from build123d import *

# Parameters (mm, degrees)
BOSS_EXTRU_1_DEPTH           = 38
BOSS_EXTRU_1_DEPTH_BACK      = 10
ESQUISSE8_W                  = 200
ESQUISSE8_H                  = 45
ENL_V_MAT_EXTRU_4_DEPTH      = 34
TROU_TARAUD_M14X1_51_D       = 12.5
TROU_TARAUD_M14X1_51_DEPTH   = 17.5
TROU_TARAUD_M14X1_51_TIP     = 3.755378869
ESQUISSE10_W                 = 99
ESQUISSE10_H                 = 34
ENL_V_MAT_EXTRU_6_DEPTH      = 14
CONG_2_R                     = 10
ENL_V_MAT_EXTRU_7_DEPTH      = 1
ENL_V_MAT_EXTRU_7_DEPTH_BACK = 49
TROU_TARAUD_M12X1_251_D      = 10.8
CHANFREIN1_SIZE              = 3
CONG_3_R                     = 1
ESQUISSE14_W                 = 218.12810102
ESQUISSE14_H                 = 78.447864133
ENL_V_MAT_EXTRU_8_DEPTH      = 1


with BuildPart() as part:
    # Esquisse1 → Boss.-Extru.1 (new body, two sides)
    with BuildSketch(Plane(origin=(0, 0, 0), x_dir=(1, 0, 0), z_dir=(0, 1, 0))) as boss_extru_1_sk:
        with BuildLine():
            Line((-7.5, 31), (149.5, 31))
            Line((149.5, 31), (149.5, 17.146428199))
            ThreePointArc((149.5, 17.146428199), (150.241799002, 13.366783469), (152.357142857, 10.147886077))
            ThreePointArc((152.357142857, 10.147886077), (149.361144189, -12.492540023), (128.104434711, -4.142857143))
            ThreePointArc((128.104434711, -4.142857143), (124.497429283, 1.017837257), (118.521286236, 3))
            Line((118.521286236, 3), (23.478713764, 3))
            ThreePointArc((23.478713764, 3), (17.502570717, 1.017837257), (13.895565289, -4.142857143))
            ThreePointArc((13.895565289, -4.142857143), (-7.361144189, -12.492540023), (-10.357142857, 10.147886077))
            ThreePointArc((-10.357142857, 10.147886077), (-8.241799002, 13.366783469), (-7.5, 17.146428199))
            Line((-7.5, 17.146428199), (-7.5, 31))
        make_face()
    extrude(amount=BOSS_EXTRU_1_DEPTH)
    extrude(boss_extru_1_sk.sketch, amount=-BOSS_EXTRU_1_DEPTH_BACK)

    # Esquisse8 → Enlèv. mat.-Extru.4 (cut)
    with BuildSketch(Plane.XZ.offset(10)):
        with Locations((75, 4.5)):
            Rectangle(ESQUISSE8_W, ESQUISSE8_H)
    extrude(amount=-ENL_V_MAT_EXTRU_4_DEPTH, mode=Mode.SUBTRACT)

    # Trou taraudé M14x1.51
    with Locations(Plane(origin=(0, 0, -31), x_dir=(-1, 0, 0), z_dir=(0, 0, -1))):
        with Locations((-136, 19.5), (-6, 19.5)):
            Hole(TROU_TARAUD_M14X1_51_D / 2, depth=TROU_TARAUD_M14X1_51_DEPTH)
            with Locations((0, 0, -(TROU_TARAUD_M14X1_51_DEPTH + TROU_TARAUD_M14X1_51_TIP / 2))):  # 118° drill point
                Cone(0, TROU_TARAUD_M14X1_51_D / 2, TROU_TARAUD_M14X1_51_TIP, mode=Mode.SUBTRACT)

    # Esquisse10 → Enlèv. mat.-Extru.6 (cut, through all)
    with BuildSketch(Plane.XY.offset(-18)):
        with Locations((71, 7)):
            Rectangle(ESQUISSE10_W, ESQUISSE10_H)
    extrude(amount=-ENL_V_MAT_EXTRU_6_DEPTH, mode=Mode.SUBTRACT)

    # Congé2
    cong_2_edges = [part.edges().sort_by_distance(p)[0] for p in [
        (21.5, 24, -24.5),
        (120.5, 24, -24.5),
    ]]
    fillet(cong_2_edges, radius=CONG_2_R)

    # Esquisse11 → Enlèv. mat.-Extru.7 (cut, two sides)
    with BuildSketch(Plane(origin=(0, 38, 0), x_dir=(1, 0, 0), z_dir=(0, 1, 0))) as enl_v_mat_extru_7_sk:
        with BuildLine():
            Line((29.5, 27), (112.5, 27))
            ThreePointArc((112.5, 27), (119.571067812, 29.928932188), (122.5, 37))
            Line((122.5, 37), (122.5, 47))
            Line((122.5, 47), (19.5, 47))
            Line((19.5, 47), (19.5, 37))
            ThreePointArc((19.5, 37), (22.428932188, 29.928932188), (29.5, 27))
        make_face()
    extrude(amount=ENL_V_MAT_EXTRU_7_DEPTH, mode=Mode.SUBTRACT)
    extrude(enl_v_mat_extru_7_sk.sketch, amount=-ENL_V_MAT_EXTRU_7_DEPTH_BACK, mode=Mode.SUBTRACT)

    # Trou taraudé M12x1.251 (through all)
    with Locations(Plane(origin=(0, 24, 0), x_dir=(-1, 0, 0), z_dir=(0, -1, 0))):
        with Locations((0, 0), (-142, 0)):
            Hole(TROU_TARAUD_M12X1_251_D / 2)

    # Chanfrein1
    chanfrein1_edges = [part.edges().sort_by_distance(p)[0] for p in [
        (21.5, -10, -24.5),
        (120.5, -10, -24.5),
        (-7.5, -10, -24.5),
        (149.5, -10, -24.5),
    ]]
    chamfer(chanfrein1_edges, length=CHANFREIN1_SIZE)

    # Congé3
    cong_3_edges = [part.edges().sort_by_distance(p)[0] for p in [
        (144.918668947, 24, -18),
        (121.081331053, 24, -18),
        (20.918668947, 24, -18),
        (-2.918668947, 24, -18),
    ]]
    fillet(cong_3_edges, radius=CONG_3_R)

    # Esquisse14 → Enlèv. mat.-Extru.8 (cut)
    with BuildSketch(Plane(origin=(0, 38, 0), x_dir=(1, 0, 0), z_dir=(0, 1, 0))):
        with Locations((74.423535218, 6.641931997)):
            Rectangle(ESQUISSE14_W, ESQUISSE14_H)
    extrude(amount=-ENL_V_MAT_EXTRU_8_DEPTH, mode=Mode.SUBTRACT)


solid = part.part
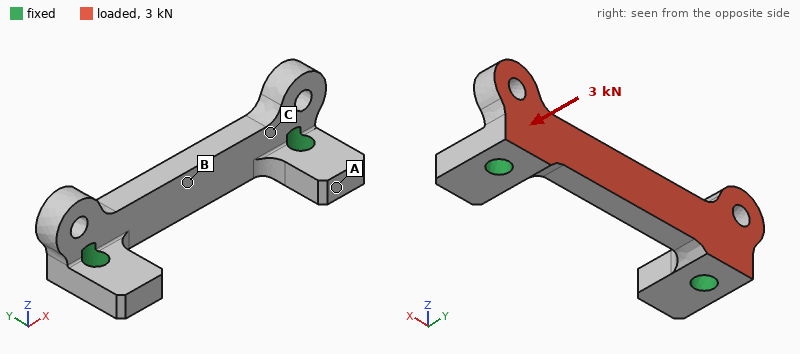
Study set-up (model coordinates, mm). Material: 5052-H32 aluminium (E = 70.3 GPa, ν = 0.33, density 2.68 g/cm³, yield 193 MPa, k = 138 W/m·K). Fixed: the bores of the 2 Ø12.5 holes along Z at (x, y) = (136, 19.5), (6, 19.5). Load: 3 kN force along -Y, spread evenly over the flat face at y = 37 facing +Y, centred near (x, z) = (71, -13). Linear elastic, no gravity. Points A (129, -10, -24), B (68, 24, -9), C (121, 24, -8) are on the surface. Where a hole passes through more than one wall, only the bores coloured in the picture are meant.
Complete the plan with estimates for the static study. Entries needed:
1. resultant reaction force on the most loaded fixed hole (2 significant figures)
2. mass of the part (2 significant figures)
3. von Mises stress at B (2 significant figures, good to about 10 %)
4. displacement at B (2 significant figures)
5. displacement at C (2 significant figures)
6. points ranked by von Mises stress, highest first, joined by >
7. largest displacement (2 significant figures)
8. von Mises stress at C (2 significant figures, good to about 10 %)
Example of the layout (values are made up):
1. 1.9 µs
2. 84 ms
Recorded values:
1. 1.6 kN
2. 230 g
3. 11 MPa
4. 28 µm
5. 7.6 µm
6. B > C > A
7. 31 µm
8. 7.2 MPa
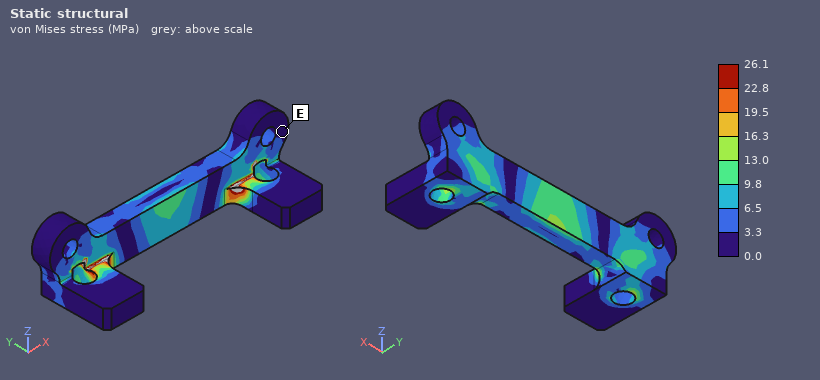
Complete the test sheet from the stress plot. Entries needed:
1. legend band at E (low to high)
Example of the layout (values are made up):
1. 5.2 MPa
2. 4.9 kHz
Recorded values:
1. 0.0 to 3.3 MPa
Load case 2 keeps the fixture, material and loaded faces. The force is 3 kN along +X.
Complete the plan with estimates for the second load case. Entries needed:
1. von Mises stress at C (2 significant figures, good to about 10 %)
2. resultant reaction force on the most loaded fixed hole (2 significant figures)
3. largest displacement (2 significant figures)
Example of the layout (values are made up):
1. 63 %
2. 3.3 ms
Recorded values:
1. 3.5 MPa
2. 1.5 kN
3. 7.5 µm
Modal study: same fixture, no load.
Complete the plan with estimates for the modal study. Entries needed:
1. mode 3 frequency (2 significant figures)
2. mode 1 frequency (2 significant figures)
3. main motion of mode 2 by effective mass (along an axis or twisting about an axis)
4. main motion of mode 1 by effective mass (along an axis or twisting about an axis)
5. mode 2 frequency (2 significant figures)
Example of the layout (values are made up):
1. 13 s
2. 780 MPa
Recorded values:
1. 8200 Hz
2. 4600 Hz
3. along Z
4. along Y
5. 6400 Hz
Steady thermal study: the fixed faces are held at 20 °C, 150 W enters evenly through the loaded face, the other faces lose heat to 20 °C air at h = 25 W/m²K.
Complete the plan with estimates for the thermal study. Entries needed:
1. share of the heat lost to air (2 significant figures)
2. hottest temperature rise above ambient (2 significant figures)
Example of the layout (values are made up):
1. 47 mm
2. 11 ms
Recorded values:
1. 3.3 %
2. 35 K
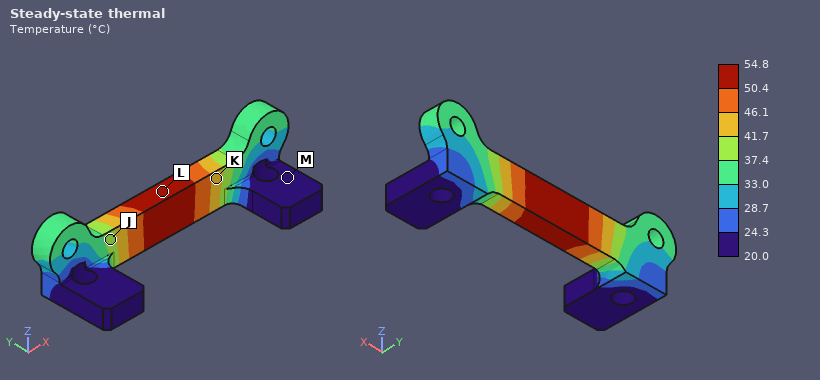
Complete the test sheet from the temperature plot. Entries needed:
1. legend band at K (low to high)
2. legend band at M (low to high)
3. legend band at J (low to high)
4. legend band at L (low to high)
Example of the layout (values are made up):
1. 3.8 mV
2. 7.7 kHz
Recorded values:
1. 41.7 to 46.1 °C
2. 20.0 to 24.3 °C
3. 37.4 to 41.7 °C
4. 50.4 to 54.8 °C
